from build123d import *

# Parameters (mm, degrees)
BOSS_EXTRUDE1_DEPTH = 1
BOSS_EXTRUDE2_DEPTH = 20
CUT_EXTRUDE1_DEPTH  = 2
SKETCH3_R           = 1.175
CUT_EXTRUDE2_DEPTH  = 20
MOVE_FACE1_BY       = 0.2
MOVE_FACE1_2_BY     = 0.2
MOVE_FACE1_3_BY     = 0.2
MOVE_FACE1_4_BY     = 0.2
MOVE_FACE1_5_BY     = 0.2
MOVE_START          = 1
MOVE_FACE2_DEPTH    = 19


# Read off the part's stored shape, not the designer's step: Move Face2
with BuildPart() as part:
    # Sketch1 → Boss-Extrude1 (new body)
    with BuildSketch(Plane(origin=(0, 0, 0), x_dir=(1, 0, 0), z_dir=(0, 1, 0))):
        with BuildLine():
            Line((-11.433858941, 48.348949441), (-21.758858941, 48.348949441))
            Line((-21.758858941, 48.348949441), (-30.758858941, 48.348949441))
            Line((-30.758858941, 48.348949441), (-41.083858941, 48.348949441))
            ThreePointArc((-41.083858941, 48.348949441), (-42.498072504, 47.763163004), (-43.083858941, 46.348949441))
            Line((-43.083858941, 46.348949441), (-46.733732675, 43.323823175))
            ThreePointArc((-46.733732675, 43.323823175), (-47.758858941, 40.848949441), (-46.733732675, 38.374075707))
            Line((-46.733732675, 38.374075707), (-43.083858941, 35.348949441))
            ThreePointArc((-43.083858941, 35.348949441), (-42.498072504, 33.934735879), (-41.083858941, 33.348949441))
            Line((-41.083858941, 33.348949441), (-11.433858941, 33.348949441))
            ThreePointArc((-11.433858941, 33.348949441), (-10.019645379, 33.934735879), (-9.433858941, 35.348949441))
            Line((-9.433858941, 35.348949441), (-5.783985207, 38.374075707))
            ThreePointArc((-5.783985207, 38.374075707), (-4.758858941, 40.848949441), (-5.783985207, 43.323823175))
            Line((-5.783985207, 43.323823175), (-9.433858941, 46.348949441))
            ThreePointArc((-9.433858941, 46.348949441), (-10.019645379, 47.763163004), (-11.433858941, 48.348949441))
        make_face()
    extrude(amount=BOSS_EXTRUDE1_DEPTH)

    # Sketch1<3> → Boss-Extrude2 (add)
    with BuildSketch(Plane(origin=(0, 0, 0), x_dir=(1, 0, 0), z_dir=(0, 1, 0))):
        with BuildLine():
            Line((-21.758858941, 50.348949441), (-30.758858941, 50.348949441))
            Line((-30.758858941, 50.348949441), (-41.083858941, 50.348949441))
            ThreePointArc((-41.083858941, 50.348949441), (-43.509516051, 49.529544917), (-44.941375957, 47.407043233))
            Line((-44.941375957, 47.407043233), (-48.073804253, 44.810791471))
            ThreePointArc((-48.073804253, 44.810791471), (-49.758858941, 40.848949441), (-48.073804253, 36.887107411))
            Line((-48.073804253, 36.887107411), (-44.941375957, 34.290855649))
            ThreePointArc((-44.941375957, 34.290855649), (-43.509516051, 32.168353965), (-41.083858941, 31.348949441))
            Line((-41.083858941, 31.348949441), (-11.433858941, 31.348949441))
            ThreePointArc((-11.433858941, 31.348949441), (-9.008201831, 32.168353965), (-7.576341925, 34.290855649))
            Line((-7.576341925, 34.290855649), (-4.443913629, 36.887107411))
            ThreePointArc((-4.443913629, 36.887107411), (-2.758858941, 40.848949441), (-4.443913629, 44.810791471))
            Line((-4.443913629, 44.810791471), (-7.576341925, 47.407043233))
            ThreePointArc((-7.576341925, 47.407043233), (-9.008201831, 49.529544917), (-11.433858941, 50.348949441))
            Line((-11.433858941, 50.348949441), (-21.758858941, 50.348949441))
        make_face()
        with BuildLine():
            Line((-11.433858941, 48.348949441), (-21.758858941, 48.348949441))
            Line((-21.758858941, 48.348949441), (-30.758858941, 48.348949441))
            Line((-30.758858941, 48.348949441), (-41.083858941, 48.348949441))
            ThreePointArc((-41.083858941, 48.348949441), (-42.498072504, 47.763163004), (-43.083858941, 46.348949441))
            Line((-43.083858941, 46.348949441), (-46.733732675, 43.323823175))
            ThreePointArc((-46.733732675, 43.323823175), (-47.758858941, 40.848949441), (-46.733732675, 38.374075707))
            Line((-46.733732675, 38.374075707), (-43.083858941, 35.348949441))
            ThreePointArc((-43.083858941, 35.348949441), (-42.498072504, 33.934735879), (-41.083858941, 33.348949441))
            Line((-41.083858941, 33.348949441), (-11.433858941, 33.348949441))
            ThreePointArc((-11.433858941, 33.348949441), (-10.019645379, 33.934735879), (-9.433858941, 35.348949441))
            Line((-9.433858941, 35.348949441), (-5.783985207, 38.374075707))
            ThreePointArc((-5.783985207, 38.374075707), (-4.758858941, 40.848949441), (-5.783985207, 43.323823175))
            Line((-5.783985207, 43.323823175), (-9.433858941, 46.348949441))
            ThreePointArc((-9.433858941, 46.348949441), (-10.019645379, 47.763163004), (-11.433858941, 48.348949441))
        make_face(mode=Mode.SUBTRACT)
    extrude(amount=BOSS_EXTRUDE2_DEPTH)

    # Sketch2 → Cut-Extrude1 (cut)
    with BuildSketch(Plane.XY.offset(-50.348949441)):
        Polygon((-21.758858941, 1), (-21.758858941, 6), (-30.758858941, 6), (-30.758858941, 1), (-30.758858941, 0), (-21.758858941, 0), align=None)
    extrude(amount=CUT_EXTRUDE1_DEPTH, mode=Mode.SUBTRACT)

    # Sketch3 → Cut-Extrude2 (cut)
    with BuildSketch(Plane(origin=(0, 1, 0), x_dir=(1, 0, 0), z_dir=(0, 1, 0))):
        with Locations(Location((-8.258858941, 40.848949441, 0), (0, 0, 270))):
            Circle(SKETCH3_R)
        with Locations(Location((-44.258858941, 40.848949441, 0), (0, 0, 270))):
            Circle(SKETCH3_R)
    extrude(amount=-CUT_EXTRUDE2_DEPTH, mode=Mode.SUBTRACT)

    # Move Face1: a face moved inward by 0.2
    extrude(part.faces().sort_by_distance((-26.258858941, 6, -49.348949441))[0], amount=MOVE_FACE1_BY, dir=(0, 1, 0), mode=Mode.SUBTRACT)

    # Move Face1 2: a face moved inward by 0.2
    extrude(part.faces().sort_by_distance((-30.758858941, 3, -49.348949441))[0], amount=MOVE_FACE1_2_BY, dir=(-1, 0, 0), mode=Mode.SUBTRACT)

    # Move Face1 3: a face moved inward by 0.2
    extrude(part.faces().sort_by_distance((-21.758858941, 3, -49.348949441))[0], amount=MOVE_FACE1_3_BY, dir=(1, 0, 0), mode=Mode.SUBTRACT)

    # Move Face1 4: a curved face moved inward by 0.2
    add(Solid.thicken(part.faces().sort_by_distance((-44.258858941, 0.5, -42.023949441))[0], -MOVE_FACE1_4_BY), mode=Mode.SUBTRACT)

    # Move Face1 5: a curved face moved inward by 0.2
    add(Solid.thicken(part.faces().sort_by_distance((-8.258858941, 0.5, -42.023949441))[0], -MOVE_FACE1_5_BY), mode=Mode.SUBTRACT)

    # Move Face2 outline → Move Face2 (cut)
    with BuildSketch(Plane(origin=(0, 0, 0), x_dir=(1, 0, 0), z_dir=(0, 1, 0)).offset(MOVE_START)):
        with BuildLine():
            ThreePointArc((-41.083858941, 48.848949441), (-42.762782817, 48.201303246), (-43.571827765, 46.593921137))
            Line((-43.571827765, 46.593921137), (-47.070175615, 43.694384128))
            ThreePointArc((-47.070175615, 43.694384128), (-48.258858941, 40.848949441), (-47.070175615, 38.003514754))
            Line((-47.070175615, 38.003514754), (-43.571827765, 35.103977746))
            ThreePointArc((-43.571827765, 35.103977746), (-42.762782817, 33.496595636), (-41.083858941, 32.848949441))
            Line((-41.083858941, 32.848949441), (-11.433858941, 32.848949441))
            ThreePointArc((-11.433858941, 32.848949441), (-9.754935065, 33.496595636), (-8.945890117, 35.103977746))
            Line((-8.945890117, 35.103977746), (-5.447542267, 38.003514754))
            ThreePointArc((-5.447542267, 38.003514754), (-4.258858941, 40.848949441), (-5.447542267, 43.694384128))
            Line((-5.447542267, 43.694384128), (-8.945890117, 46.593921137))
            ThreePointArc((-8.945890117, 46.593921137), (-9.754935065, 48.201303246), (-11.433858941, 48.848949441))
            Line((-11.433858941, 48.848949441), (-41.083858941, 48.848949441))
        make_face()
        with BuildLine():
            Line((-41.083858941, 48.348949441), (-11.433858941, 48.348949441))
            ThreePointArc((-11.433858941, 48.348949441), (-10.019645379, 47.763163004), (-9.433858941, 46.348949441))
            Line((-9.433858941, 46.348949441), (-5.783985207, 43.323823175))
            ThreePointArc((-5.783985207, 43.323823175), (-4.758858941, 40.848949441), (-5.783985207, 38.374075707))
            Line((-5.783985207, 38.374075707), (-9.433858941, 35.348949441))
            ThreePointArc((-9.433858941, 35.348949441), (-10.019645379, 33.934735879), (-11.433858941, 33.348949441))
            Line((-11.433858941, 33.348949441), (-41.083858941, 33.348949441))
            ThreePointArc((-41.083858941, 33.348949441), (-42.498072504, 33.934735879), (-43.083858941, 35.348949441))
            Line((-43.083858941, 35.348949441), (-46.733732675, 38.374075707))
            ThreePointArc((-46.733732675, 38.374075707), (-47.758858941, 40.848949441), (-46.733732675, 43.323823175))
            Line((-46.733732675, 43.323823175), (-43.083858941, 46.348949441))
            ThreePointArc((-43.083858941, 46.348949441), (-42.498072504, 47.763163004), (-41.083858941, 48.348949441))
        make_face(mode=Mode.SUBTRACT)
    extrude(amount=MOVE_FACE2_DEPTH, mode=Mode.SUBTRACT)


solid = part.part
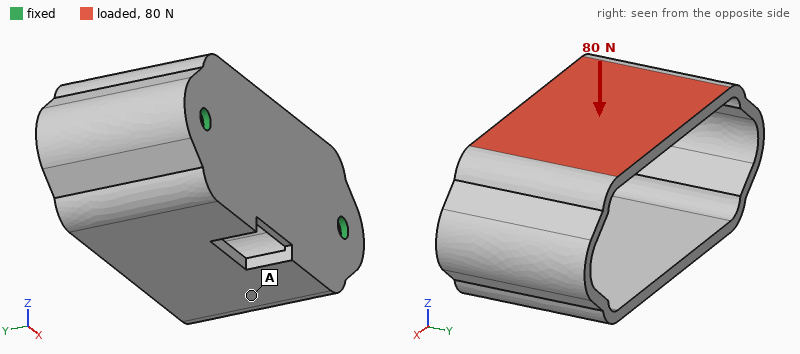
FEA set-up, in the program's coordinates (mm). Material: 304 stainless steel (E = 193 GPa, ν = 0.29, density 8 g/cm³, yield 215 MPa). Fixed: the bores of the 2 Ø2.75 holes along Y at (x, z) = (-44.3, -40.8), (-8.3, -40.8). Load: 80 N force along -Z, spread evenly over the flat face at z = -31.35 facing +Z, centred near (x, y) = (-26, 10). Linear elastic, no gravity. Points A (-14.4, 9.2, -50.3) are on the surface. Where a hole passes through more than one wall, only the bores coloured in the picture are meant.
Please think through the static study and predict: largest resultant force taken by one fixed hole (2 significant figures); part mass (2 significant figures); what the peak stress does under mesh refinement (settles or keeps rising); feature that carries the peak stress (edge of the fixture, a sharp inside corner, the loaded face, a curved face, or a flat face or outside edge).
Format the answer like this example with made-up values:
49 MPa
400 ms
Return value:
41 N
30 g
keeps rising
edge of the fixture
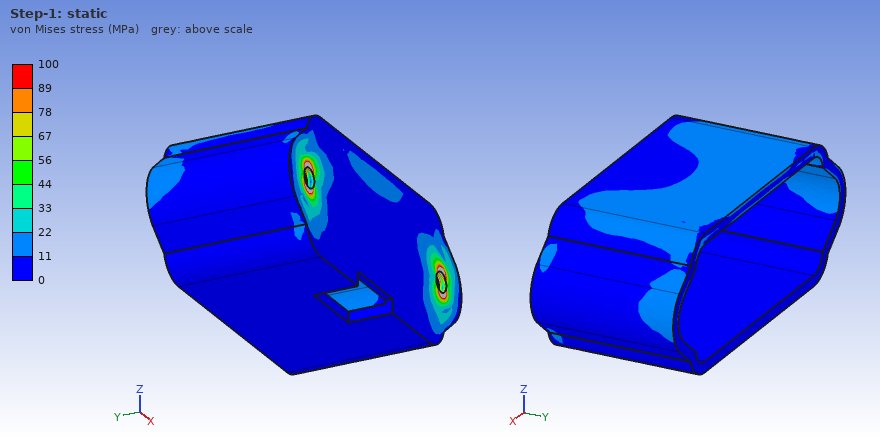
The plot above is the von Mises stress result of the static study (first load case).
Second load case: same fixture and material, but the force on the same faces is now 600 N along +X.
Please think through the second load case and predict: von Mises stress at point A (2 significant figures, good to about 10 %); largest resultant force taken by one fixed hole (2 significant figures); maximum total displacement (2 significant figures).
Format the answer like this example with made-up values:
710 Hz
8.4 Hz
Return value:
14 MPa
370 N
31 µm
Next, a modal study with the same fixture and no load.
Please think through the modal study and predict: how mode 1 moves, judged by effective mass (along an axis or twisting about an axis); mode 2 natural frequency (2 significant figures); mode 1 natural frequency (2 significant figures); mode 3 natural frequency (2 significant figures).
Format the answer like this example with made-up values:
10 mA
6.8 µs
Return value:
along Z
3800 Hz
1800 Hz
4200 Hz
